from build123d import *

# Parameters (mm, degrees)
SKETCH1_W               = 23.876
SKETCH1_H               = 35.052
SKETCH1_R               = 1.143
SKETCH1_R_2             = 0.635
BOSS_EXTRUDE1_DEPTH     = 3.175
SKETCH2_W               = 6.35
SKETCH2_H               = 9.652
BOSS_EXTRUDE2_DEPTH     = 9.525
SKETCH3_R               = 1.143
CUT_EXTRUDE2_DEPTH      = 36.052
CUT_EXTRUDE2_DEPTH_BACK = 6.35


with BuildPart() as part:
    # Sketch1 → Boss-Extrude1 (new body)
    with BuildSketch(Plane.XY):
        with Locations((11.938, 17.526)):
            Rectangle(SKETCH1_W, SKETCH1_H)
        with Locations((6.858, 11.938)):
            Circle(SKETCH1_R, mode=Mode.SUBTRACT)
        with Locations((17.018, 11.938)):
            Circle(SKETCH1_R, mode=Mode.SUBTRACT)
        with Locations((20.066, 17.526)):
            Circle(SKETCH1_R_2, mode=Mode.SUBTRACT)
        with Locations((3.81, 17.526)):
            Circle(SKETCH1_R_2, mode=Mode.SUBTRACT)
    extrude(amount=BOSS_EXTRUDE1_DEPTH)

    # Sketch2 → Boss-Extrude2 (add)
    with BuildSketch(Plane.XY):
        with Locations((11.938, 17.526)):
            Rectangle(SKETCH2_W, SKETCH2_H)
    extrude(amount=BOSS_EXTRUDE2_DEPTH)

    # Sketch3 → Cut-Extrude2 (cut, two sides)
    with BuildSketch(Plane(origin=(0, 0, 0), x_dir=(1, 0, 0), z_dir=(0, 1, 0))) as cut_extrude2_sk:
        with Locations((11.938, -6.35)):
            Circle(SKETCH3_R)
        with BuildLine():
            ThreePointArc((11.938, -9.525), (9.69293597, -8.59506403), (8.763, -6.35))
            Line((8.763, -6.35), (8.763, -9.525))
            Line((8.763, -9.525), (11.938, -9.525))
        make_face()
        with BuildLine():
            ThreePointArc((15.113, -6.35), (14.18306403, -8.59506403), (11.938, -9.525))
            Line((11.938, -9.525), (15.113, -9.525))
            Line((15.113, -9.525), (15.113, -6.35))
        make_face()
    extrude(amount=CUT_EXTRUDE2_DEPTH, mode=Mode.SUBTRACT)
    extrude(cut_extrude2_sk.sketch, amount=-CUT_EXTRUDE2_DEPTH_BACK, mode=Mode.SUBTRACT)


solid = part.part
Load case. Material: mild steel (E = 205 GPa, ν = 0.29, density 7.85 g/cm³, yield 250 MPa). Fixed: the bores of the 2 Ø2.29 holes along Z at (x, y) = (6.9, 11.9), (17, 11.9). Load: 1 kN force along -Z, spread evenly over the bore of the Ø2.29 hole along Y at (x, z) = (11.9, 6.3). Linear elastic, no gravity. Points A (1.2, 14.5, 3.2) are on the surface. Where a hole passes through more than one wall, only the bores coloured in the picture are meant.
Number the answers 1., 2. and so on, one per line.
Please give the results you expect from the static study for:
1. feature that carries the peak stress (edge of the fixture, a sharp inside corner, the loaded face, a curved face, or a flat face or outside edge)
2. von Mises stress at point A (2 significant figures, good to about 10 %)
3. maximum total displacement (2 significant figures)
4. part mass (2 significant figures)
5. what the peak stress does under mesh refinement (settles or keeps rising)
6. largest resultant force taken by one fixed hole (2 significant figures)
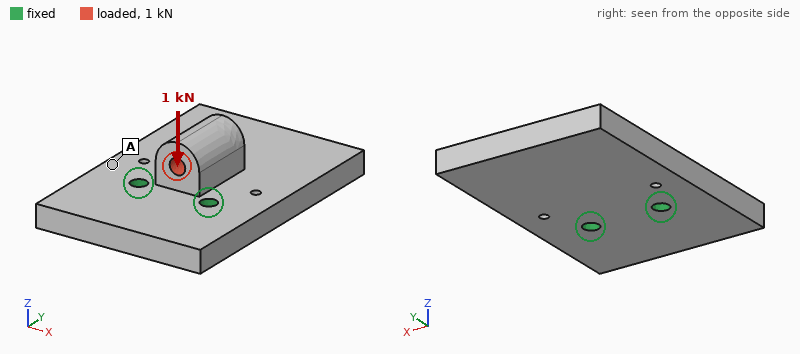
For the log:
1. edge of the fixture
2. 46 MPa
3. 33 µm
4. 23 g
5. keeps rising
6. 500 N
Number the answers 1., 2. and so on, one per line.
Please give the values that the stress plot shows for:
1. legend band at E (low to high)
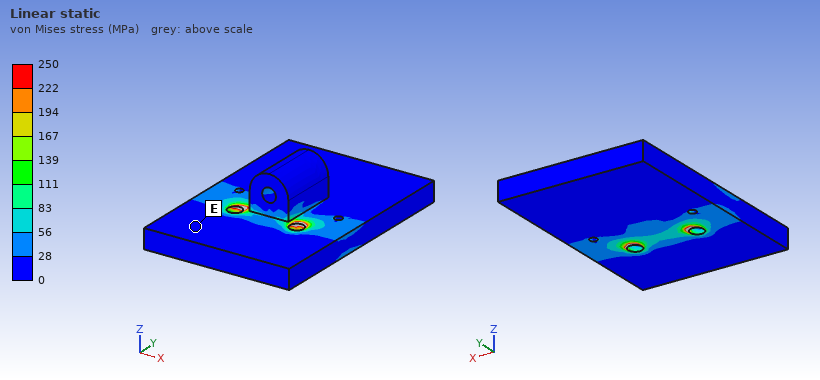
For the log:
1. 0 to 28 MPa
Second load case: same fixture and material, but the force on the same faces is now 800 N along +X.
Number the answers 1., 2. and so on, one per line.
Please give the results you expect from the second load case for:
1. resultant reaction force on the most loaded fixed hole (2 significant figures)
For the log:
1. 670 N
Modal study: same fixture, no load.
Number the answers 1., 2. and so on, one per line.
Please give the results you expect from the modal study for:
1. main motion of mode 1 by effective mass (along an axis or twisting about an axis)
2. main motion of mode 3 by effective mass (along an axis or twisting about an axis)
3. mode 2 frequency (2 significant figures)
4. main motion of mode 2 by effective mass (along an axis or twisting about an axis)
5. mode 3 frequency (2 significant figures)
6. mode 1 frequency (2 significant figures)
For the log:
1. along Z
2. along Z
3. 12 kHz
4. twisting about Y
5. 17 kHz
6. 5200 Hz
